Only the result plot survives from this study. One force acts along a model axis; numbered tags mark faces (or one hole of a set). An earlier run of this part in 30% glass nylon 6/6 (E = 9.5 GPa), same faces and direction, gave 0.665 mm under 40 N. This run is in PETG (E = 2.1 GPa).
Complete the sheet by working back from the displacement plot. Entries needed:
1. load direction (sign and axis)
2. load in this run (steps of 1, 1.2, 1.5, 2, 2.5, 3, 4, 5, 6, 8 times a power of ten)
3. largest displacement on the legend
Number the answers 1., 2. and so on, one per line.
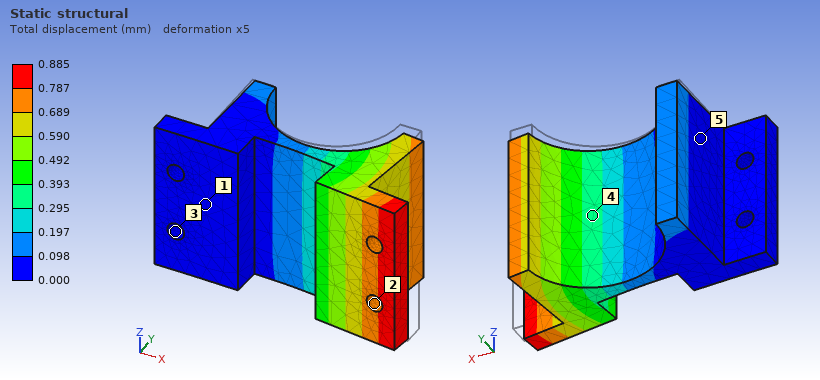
1. -Y
2. 12 N
3. 0.885 mm
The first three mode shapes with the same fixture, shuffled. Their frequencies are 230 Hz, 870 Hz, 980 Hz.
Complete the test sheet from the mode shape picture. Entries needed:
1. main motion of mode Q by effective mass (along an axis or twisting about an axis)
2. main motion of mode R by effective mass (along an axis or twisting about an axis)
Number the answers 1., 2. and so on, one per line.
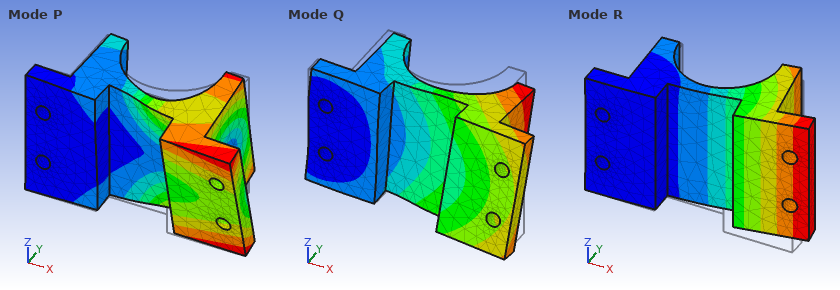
1. along Z
2. along Y
